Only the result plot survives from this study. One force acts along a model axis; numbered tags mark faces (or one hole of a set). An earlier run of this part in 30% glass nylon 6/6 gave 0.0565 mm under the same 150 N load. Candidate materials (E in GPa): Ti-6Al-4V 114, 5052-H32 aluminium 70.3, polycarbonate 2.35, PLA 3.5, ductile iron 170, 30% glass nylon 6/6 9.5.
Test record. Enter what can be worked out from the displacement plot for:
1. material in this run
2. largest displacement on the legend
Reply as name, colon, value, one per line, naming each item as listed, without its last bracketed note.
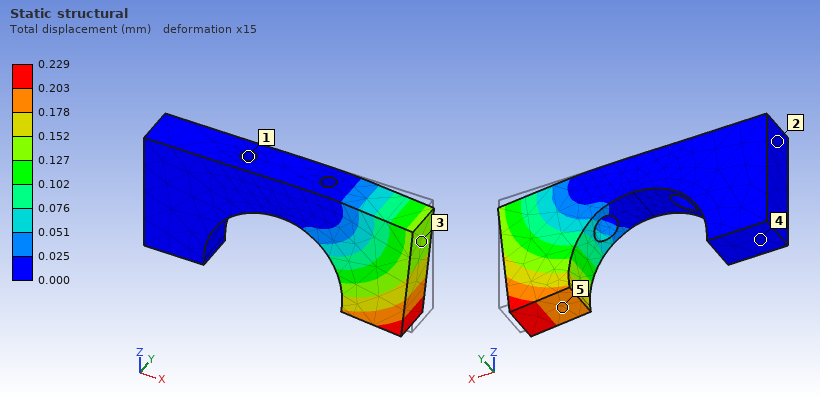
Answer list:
material in this run: polycarbonate
largest displacement on the legend: 0.229 mm
